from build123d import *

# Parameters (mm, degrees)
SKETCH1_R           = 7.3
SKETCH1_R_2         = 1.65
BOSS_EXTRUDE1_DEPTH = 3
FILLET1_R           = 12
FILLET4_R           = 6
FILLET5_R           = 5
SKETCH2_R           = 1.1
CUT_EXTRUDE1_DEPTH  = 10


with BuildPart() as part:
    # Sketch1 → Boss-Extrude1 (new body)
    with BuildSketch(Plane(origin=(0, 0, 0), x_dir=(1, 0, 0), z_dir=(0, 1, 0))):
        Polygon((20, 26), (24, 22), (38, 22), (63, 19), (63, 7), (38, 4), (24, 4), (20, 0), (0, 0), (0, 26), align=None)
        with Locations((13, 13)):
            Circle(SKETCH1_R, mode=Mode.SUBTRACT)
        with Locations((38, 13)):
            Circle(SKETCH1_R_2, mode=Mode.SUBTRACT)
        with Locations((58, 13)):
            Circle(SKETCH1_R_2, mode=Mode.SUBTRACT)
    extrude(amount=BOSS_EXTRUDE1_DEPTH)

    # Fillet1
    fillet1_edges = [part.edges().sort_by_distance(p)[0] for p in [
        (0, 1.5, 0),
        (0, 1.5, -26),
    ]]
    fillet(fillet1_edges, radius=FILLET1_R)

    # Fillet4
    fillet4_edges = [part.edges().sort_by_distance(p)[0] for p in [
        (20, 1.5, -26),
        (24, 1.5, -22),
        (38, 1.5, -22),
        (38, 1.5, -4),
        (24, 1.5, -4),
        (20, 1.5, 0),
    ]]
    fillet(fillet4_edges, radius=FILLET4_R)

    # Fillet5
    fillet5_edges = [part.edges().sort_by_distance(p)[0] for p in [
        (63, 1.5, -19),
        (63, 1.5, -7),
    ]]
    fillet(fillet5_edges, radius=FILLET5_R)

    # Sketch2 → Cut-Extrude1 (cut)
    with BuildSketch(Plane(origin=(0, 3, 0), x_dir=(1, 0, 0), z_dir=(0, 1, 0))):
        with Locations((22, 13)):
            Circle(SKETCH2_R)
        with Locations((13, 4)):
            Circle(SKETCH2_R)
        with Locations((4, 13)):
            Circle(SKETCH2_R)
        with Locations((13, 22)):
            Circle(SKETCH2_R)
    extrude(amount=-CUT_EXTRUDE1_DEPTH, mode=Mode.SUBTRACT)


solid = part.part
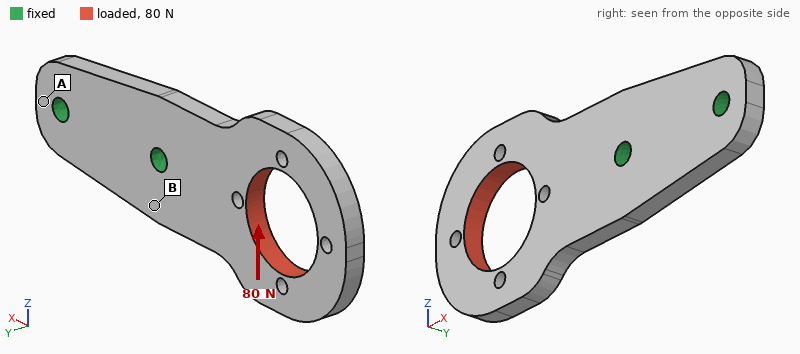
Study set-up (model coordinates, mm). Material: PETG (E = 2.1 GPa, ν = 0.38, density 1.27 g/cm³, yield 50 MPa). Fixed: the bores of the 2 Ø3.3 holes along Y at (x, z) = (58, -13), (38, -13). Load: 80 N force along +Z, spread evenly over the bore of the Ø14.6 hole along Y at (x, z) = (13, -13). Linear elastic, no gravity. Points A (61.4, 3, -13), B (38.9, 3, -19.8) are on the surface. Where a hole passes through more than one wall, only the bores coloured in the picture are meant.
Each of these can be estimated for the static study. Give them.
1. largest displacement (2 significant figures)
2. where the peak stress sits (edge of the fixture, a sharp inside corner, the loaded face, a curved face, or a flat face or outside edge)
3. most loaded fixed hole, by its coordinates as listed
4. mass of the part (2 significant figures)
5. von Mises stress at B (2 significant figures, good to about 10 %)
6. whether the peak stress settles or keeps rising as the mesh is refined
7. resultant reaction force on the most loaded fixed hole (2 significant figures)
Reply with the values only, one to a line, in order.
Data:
0.69 mm
edge of the fixture
(38, -13)
3.7 g
8.2 MPa
keeps rising
150 N
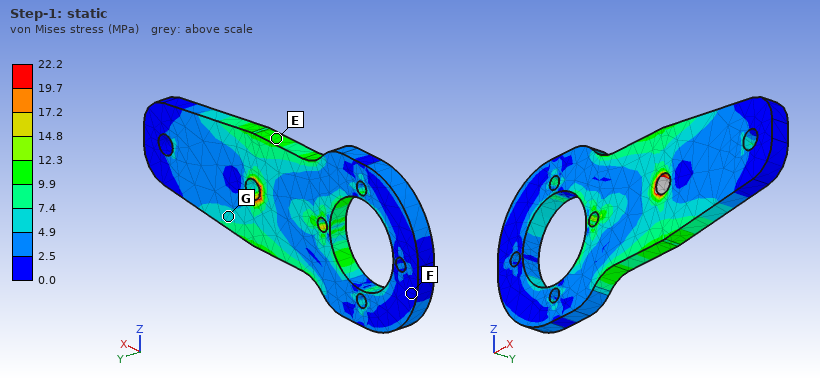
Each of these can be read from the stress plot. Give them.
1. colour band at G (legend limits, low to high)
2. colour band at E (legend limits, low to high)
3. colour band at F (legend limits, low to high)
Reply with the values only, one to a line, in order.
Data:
4.9 to 7.4 MPa
9.9 to 12.3 MPa
0.0 to 2.5 MPa
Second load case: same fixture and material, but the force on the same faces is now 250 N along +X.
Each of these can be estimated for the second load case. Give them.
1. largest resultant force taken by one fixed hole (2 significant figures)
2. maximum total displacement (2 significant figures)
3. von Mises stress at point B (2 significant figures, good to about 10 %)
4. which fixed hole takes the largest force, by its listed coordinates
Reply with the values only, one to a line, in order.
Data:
210 N
0.18 mm
2.7 MPa
(38, -13)
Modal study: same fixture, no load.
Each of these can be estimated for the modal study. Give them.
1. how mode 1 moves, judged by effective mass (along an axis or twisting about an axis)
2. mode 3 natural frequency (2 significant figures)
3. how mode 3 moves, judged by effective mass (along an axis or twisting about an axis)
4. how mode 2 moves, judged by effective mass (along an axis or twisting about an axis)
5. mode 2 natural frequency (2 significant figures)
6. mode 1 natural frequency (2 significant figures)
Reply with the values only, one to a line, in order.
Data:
along Y
1600 Hz
along Z
twisting about X
1100 Hz
470 Hz
